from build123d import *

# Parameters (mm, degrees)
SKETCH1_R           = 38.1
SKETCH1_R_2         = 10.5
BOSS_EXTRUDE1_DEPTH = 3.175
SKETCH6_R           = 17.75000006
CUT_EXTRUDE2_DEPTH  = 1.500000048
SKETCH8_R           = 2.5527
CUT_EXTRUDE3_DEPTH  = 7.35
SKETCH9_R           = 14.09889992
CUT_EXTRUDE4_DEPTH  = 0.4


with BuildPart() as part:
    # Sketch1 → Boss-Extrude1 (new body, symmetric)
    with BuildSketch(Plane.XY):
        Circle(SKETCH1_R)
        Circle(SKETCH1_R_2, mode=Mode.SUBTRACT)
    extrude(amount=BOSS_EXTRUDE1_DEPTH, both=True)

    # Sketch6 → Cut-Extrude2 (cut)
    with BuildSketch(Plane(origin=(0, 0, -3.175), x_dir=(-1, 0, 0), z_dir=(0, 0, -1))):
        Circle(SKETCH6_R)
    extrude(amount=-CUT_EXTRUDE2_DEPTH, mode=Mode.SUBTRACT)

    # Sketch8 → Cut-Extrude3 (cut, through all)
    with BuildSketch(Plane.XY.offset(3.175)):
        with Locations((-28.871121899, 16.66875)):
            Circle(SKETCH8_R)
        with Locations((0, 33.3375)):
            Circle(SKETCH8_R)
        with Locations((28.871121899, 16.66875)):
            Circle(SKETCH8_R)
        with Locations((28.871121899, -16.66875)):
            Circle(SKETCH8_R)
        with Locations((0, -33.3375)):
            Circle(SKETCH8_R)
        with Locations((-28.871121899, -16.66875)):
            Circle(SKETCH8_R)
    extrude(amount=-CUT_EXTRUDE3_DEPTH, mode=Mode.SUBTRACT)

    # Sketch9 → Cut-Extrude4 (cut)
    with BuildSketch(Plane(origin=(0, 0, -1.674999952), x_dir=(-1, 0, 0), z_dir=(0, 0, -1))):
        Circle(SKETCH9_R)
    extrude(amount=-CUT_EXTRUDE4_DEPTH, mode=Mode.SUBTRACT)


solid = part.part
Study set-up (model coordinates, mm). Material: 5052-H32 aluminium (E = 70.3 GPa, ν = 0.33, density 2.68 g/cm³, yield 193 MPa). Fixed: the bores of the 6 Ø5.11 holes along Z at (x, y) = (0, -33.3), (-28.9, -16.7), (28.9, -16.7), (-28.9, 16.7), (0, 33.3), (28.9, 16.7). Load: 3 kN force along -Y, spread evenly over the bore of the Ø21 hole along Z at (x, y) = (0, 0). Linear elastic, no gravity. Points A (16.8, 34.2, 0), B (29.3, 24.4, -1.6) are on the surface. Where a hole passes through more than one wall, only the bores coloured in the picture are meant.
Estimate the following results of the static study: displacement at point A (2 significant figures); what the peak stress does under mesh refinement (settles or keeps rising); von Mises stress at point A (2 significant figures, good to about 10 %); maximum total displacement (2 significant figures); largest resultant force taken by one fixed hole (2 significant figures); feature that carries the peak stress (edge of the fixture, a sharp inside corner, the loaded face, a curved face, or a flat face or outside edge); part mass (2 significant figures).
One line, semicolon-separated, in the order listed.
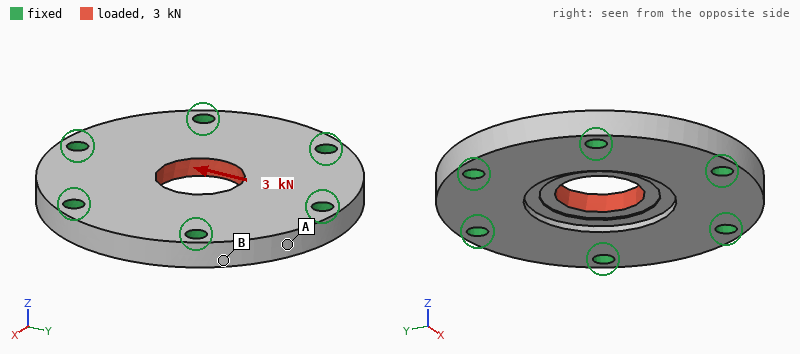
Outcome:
1.1 µm; keeps rising; 3.6 MPa; 3.5 µm; 750 N; edge of the fixture; 67 g
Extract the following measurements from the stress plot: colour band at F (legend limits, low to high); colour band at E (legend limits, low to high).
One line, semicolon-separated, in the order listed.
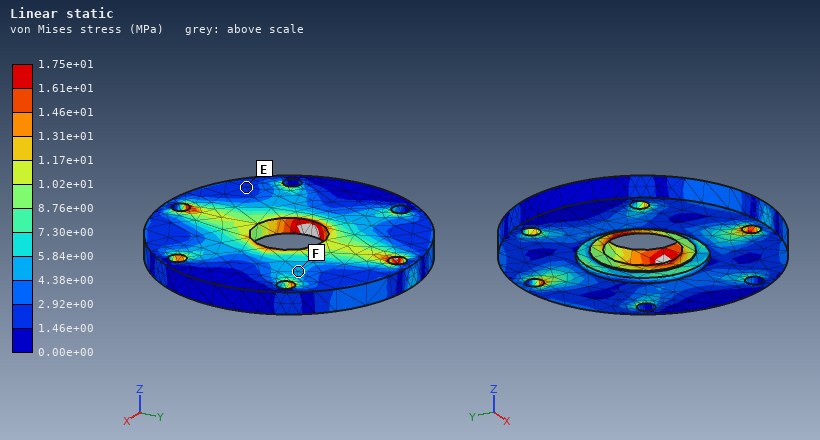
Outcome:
4.38e+00 to 5.84e+00 MPa; 1.46e+00 to 2.92e+00 MPa
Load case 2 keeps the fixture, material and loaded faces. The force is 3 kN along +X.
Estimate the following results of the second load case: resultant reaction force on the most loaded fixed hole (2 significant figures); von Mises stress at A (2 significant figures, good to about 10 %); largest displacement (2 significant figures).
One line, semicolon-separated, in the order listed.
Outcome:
660 N; 1.9 MPa; 3.6 µm
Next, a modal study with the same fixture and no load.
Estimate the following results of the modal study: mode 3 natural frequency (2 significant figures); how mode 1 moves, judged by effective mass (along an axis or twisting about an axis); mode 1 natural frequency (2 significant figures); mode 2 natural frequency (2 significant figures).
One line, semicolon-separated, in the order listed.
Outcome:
19 kHz; along Z; 13 kHz; 19 kHz
